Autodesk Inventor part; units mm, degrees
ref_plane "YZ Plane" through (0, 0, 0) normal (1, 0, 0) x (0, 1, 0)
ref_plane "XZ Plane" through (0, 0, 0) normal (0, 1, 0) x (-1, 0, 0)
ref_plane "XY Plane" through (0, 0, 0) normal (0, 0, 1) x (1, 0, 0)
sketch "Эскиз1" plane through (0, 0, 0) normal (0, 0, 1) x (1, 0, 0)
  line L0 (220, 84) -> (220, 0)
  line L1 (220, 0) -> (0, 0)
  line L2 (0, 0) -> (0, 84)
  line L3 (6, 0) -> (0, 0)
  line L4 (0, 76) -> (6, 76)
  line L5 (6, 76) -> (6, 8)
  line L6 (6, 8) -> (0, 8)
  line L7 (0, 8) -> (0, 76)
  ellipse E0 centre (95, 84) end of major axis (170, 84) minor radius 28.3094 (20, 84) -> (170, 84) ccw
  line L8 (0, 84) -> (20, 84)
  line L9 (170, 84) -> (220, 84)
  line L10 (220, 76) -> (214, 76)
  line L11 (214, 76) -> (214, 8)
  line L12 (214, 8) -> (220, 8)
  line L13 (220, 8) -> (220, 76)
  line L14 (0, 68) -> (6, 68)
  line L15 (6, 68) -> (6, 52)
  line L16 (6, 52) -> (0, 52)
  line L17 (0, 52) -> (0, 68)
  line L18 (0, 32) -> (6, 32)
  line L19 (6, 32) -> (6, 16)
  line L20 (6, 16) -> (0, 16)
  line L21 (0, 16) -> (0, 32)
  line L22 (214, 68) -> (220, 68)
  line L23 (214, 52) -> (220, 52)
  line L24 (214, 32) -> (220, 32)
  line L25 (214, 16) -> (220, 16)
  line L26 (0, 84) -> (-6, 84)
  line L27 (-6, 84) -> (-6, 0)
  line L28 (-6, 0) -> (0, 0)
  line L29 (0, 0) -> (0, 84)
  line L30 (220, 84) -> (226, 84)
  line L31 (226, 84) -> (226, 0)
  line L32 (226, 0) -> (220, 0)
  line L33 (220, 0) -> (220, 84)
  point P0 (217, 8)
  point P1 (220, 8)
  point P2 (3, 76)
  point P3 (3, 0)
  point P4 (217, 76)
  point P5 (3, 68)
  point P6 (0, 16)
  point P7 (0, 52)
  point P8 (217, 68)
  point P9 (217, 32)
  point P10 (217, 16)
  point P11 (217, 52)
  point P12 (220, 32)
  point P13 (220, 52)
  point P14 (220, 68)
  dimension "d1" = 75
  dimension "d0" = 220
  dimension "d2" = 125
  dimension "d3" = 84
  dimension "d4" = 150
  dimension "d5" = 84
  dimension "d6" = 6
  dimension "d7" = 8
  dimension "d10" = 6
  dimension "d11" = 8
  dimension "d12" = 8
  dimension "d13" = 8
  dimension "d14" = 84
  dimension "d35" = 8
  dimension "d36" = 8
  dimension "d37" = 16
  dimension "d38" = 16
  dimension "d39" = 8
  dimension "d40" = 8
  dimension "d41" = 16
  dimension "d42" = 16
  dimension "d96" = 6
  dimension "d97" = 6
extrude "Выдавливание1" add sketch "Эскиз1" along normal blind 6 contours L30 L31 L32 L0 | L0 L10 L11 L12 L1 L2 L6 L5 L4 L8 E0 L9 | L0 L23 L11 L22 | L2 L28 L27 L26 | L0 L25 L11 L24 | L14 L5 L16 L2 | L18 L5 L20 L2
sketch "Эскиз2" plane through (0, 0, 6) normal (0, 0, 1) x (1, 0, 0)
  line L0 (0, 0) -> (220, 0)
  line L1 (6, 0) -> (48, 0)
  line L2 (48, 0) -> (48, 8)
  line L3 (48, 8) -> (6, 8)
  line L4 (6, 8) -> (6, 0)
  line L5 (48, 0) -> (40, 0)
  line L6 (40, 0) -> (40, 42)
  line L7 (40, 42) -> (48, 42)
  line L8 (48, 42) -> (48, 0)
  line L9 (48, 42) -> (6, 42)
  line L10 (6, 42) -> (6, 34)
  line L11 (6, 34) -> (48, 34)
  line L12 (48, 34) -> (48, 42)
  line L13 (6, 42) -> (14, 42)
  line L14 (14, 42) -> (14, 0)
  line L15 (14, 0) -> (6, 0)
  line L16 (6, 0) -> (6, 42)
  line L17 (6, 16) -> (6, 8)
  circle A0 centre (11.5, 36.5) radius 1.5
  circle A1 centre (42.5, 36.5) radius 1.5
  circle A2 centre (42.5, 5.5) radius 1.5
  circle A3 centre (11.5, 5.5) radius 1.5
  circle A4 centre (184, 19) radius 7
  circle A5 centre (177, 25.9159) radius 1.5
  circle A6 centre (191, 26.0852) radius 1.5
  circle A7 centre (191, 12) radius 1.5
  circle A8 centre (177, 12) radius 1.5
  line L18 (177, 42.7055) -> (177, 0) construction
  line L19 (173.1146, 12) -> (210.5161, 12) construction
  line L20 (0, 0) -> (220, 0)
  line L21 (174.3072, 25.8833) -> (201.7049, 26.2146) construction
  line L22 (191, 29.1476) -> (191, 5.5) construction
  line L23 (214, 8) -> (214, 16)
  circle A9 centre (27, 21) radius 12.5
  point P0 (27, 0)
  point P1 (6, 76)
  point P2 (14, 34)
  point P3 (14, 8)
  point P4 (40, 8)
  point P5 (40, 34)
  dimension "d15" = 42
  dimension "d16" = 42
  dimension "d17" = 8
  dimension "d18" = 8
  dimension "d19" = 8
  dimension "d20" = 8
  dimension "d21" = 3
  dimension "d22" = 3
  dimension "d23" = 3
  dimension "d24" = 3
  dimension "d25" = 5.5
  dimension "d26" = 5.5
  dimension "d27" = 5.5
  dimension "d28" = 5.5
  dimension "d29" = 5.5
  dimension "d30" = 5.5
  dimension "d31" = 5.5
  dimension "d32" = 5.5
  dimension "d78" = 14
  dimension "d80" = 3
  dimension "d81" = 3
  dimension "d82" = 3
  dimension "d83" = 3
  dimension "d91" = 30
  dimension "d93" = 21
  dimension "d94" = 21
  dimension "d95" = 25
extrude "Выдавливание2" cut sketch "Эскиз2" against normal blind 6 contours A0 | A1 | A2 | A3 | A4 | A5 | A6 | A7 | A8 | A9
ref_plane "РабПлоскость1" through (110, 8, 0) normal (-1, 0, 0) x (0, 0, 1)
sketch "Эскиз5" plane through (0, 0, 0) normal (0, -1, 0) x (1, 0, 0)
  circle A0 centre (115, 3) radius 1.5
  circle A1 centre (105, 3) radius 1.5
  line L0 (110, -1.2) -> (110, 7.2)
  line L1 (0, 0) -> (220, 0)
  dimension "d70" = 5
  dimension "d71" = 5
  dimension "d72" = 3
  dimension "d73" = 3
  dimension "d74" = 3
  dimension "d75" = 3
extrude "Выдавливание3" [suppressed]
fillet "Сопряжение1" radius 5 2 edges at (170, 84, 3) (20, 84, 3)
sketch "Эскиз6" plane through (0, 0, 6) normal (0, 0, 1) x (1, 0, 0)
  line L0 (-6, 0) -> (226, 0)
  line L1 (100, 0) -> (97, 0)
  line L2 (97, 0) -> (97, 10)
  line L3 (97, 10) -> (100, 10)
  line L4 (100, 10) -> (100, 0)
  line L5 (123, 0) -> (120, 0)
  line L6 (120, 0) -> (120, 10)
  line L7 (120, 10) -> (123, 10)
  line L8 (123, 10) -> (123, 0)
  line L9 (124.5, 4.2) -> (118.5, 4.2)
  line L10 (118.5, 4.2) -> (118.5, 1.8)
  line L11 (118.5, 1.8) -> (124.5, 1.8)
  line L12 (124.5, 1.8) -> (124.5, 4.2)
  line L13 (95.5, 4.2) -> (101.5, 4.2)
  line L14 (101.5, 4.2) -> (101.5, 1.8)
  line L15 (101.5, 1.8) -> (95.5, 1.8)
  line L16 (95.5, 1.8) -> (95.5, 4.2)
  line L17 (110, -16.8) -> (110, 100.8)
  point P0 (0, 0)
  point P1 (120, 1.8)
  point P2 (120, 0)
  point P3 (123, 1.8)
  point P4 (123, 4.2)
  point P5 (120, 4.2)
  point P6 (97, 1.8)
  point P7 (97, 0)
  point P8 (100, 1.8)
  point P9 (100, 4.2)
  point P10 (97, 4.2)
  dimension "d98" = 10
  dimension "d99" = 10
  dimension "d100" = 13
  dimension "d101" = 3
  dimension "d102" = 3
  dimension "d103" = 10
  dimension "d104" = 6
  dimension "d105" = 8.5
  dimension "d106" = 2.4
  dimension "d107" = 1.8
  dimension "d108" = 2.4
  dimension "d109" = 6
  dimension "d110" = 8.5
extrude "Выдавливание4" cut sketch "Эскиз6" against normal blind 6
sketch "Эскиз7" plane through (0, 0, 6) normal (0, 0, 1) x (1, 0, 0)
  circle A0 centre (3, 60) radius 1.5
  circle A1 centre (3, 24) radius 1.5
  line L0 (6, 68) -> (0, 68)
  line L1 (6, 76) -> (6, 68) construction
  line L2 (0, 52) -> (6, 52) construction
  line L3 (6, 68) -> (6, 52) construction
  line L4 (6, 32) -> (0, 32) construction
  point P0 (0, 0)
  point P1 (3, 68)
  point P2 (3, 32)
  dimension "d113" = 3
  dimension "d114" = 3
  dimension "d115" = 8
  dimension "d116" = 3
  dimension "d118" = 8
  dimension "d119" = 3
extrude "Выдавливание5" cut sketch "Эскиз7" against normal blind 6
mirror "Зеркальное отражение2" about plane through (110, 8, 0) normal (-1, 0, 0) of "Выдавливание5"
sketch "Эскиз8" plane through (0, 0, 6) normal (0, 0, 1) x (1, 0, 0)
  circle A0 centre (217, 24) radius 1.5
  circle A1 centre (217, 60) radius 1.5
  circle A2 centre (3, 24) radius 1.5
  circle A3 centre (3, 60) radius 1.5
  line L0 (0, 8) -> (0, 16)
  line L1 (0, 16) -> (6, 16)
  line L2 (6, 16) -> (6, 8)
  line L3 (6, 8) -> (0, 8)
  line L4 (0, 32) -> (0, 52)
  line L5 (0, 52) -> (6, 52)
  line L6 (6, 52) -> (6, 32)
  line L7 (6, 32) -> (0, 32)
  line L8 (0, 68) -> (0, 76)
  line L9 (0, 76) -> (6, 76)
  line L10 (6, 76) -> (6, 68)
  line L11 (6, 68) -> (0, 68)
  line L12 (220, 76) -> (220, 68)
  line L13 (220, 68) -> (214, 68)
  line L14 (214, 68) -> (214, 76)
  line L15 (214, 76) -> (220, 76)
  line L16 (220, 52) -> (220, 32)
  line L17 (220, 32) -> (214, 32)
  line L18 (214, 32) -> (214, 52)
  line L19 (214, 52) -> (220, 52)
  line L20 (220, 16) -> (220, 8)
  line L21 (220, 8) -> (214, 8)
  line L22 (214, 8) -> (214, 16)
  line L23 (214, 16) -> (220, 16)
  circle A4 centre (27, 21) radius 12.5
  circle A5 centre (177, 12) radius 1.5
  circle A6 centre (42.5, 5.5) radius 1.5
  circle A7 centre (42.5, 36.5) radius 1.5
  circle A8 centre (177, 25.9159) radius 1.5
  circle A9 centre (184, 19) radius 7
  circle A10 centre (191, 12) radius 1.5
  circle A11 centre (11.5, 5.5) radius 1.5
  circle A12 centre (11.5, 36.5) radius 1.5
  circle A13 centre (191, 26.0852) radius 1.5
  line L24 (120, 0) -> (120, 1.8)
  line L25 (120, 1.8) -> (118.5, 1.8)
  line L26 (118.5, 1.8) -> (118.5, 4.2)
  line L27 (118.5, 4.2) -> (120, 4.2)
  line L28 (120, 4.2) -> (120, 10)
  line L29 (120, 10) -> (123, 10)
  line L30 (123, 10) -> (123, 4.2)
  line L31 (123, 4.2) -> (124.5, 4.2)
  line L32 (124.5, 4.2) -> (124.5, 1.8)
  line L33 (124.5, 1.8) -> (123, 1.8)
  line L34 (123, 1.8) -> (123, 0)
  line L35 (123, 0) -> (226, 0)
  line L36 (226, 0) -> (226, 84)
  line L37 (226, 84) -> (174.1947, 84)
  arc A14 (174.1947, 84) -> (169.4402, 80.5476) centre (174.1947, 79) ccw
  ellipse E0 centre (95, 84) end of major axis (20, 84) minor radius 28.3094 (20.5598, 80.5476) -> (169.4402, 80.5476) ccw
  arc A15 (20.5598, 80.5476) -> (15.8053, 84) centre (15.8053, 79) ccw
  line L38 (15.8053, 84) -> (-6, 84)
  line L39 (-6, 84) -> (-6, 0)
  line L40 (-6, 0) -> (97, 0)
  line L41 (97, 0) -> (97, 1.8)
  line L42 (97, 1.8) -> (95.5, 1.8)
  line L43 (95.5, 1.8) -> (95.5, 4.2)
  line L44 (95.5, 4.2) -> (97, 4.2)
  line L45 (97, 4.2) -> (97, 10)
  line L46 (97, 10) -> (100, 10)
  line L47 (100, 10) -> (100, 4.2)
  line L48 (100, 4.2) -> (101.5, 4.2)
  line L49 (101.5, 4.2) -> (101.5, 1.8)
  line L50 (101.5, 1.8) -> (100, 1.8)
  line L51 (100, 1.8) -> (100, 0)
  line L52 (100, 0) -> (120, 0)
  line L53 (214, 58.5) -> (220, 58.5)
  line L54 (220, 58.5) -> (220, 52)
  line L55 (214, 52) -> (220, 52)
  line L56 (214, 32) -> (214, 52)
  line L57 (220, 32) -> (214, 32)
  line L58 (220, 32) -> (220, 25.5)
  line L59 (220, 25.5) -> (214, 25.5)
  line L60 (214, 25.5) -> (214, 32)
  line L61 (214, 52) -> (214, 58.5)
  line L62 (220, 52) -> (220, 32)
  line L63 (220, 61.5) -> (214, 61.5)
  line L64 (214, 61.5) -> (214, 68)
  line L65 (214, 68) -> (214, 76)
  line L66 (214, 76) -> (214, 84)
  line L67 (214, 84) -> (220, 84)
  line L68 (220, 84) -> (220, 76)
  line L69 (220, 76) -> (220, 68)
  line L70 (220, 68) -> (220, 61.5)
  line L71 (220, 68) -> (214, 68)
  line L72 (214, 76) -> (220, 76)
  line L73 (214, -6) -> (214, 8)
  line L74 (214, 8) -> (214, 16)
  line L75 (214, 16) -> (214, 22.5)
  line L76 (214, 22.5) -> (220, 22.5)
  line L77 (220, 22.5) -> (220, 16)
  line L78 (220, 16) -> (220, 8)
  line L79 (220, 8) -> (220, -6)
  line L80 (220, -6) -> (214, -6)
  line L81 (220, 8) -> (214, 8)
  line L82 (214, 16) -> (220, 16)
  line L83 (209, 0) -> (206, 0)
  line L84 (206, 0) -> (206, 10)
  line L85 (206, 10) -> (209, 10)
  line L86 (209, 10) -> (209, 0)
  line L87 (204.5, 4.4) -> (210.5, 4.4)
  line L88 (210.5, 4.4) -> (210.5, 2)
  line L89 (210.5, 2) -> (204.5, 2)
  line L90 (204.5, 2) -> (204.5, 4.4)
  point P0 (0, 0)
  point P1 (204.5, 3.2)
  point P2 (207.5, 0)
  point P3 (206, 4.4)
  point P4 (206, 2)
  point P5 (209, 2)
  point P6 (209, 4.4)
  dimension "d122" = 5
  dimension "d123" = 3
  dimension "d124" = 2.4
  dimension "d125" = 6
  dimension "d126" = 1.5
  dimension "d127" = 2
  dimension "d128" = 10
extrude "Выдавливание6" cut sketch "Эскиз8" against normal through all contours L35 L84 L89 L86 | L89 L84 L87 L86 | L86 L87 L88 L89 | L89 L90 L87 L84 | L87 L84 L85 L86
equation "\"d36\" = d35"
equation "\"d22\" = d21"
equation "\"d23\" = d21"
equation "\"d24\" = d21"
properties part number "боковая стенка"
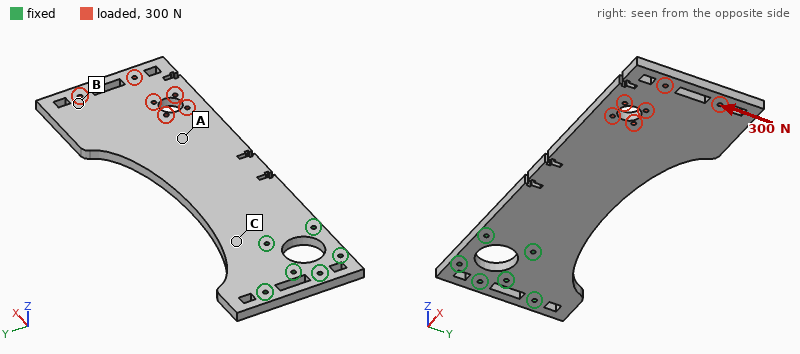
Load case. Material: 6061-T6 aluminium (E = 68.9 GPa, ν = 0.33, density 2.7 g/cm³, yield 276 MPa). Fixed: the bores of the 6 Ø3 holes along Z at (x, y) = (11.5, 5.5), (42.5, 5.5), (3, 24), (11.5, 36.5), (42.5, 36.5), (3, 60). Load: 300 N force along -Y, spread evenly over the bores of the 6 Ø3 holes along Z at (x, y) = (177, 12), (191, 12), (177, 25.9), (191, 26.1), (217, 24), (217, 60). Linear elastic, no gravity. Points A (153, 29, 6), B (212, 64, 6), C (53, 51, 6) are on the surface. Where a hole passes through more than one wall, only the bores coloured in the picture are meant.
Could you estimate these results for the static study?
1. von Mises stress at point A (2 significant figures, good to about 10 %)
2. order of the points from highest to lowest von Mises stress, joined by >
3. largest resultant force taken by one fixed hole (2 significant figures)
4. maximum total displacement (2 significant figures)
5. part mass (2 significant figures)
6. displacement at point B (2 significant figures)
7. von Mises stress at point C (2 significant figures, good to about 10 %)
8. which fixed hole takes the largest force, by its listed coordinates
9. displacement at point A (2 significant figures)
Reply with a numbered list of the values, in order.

1. 2.8 MPa
2. C > A > B
3. 1.0 kN
4. 0.11 mm
5. 240 g
6. 0.094 mm
7. 6.5 MPa
8. (42.5, 5.5)
9. 0.048 mm
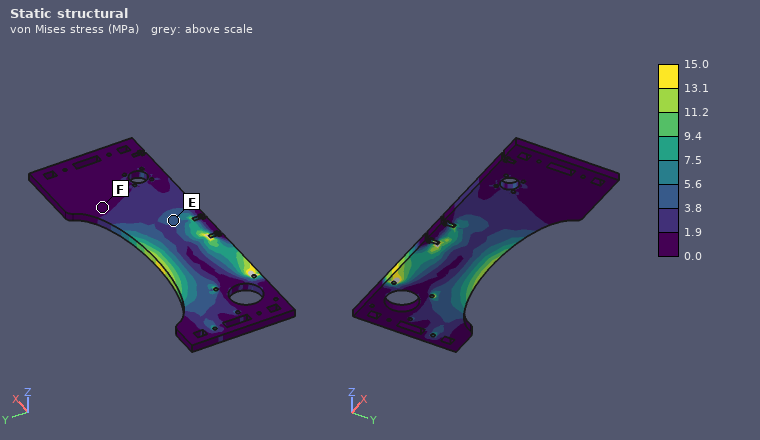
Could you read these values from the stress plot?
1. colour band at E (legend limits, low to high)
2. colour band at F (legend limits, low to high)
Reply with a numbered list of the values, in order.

1. 3.8 to 5.6 MPa
2. 0.0 to 1.9 MPa
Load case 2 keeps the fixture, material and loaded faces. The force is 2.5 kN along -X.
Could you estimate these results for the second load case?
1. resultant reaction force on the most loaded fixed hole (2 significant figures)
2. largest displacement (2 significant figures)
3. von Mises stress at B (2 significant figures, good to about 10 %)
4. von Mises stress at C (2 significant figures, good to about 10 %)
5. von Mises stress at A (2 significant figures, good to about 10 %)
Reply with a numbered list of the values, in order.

1. 1.1 kN
2. 44 µm
3. 3.7 MPa
4. 4.6 MPa
5. 8.1 MPa
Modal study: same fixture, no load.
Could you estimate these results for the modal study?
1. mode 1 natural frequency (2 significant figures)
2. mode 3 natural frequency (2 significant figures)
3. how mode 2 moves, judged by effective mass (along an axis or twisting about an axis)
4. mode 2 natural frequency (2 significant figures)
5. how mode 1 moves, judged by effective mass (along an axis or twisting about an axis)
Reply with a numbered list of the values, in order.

1. 120 Hz
2. 860 Hz
3. twisting about X
4. 580 Hz
5. along Z
